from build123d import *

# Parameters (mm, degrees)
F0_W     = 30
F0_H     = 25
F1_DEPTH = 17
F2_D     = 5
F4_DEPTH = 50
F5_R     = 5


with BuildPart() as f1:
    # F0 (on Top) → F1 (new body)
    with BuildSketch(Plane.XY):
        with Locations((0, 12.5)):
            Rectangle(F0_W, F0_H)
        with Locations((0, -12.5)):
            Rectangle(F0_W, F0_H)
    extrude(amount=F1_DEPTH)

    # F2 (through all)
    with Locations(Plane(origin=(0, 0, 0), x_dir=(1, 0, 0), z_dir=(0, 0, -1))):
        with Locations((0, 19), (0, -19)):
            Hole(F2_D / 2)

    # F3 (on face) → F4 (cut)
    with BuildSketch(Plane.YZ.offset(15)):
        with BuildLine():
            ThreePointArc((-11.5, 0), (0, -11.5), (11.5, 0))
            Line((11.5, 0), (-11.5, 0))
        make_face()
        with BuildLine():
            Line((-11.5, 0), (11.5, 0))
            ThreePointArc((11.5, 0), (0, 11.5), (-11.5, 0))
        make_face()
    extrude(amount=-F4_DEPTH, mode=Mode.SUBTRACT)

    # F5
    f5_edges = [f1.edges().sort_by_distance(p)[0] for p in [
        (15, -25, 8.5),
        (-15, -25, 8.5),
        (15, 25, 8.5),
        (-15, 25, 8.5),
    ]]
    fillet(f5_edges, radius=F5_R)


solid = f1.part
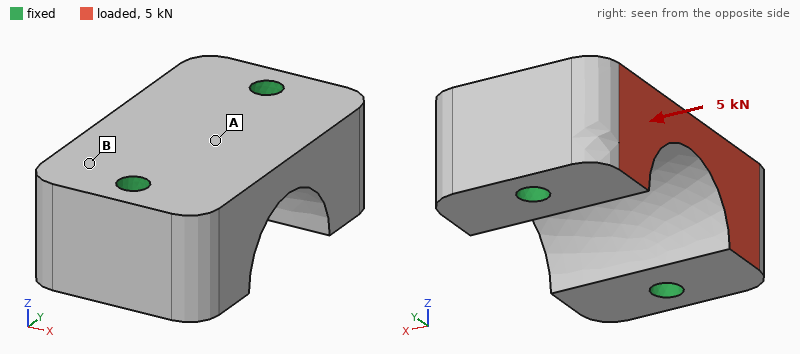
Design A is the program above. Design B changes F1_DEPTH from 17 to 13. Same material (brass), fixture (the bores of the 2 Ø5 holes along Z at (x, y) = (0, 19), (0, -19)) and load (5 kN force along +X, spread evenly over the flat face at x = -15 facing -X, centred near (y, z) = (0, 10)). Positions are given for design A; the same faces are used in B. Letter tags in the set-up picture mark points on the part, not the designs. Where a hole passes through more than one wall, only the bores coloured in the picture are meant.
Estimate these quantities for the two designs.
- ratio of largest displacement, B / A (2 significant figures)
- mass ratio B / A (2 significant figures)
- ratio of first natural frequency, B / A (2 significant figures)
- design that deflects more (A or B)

1.9
0.68
0.92
B
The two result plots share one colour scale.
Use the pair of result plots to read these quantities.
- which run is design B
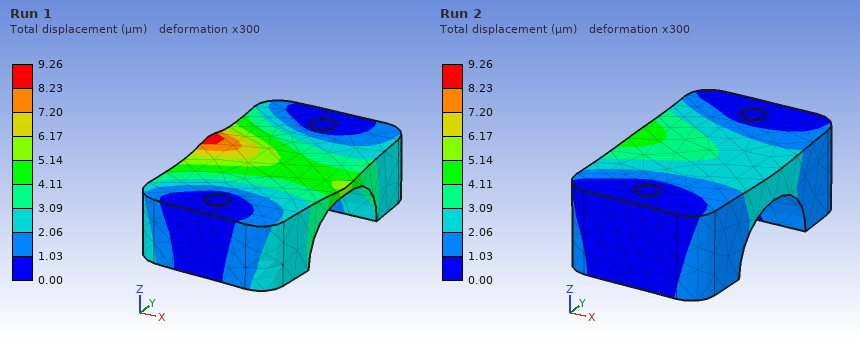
Run 1
